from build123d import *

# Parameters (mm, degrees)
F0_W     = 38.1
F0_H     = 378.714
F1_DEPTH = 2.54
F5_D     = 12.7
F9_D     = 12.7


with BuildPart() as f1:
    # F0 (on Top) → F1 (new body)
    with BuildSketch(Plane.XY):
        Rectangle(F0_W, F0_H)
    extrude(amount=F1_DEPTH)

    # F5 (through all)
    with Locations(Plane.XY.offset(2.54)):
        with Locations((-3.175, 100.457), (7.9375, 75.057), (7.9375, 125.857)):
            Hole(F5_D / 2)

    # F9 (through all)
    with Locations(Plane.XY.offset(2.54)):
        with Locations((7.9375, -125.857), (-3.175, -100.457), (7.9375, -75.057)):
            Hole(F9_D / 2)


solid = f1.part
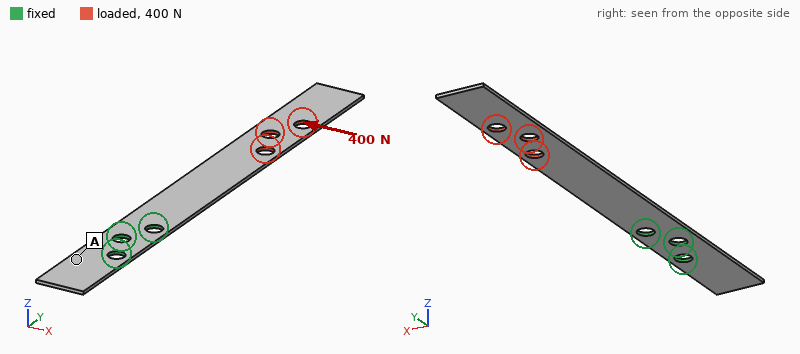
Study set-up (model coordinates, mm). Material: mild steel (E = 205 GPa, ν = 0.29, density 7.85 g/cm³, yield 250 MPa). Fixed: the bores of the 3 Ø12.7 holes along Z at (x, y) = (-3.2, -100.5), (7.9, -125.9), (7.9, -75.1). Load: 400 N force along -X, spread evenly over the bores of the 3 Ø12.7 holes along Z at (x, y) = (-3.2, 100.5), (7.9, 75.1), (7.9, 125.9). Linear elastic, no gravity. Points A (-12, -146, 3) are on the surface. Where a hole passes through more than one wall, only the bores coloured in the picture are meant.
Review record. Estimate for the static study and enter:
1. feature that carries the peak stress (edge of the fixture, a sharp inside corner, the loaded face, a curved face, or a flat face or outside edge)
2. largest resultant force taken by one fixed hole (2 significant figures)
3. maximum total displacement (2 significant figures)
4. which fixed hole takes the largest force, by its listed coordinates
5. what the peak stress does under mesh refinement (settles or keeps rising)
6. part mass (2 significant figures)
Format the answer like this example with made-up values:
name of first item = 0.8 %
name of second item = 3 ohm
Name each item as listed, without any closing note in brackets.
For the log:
feature that carries the peak stress = edge of the fixture
largest resultant force taken by one fixed hole = 2.0 kN
maximum total displacement = 0.60 mm
which fixed hole takes the largest force, by its listed coordinates = (7.9, -75.1)
what the peak stress does under mesh refinement = keeps rising
part mass = 270 g
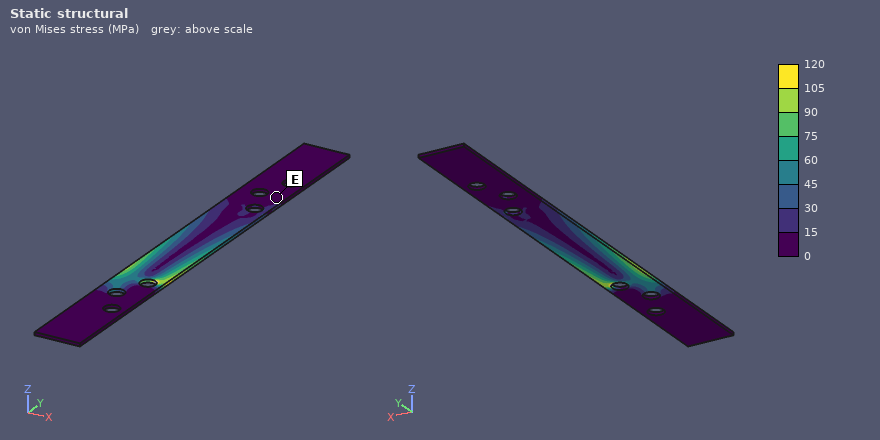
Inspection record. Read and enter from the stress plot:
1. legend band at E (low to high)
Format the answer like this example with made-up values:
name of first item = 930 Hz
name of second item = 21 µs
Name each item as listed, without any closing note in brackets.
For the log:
legend band at E = 0 to 15 MPa
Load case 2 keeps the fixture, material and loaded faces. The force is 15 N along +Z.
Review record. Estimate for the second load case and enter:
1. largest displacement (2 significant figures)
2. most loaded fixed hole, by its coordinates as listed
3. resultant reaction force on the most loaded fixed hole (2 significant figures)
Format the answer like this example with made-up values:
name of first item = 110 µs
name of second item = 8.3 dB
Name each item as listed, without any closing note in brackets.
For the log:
largest displacement = 4.2 mm
most loaded fixed hole, by its coordinates as listed = (7.9, -75.1)
resultant reaction force on the most loaded fixed hole = 38 N
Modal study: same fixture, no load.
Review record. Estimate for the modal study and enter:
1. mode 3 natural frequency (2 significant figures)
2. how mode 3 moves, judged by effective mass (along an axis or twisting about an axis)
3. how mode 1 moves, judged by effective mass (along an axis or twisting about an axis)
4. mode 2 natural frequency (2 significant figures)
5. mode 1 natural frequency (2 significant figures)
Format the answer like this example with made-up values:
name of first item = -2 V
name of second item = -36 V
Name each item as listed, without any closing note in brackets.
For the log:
mode 3 natural frequency = 400 Hz
how mode 3 moves, judged by effective mass = twisting about Y
how mode 1 moves, judged by effective mass = along Z
mode 2 natural frequency = 190 Hz
mode 1 natural frequency = 32 Hz
